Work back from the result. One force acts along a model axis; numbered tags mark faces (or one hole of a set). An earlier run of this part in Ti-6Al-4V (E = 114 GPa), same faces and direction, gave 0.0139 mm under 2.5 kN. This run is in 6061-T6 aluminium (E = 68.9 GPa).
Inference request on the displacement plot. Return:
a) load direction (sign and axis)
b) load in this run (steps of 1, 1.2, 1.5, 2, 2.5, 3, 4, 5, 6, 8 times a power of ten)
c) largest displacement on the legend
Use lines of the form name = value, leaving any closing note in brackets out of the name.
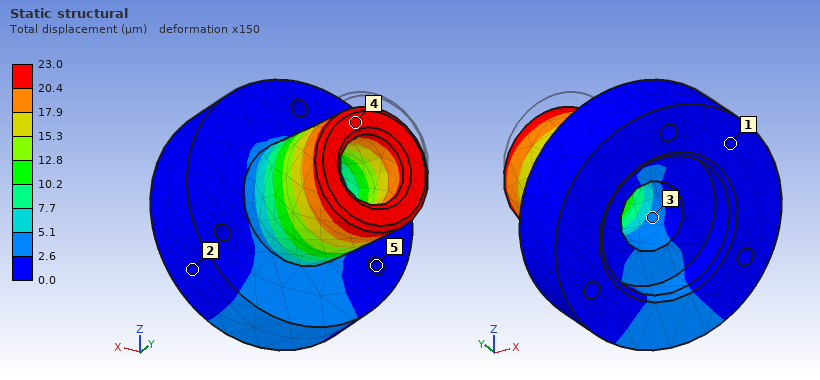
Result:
load direction = -Z
load in this run = 2.5 kN
largest displacement on the legend = 23.0 µm
